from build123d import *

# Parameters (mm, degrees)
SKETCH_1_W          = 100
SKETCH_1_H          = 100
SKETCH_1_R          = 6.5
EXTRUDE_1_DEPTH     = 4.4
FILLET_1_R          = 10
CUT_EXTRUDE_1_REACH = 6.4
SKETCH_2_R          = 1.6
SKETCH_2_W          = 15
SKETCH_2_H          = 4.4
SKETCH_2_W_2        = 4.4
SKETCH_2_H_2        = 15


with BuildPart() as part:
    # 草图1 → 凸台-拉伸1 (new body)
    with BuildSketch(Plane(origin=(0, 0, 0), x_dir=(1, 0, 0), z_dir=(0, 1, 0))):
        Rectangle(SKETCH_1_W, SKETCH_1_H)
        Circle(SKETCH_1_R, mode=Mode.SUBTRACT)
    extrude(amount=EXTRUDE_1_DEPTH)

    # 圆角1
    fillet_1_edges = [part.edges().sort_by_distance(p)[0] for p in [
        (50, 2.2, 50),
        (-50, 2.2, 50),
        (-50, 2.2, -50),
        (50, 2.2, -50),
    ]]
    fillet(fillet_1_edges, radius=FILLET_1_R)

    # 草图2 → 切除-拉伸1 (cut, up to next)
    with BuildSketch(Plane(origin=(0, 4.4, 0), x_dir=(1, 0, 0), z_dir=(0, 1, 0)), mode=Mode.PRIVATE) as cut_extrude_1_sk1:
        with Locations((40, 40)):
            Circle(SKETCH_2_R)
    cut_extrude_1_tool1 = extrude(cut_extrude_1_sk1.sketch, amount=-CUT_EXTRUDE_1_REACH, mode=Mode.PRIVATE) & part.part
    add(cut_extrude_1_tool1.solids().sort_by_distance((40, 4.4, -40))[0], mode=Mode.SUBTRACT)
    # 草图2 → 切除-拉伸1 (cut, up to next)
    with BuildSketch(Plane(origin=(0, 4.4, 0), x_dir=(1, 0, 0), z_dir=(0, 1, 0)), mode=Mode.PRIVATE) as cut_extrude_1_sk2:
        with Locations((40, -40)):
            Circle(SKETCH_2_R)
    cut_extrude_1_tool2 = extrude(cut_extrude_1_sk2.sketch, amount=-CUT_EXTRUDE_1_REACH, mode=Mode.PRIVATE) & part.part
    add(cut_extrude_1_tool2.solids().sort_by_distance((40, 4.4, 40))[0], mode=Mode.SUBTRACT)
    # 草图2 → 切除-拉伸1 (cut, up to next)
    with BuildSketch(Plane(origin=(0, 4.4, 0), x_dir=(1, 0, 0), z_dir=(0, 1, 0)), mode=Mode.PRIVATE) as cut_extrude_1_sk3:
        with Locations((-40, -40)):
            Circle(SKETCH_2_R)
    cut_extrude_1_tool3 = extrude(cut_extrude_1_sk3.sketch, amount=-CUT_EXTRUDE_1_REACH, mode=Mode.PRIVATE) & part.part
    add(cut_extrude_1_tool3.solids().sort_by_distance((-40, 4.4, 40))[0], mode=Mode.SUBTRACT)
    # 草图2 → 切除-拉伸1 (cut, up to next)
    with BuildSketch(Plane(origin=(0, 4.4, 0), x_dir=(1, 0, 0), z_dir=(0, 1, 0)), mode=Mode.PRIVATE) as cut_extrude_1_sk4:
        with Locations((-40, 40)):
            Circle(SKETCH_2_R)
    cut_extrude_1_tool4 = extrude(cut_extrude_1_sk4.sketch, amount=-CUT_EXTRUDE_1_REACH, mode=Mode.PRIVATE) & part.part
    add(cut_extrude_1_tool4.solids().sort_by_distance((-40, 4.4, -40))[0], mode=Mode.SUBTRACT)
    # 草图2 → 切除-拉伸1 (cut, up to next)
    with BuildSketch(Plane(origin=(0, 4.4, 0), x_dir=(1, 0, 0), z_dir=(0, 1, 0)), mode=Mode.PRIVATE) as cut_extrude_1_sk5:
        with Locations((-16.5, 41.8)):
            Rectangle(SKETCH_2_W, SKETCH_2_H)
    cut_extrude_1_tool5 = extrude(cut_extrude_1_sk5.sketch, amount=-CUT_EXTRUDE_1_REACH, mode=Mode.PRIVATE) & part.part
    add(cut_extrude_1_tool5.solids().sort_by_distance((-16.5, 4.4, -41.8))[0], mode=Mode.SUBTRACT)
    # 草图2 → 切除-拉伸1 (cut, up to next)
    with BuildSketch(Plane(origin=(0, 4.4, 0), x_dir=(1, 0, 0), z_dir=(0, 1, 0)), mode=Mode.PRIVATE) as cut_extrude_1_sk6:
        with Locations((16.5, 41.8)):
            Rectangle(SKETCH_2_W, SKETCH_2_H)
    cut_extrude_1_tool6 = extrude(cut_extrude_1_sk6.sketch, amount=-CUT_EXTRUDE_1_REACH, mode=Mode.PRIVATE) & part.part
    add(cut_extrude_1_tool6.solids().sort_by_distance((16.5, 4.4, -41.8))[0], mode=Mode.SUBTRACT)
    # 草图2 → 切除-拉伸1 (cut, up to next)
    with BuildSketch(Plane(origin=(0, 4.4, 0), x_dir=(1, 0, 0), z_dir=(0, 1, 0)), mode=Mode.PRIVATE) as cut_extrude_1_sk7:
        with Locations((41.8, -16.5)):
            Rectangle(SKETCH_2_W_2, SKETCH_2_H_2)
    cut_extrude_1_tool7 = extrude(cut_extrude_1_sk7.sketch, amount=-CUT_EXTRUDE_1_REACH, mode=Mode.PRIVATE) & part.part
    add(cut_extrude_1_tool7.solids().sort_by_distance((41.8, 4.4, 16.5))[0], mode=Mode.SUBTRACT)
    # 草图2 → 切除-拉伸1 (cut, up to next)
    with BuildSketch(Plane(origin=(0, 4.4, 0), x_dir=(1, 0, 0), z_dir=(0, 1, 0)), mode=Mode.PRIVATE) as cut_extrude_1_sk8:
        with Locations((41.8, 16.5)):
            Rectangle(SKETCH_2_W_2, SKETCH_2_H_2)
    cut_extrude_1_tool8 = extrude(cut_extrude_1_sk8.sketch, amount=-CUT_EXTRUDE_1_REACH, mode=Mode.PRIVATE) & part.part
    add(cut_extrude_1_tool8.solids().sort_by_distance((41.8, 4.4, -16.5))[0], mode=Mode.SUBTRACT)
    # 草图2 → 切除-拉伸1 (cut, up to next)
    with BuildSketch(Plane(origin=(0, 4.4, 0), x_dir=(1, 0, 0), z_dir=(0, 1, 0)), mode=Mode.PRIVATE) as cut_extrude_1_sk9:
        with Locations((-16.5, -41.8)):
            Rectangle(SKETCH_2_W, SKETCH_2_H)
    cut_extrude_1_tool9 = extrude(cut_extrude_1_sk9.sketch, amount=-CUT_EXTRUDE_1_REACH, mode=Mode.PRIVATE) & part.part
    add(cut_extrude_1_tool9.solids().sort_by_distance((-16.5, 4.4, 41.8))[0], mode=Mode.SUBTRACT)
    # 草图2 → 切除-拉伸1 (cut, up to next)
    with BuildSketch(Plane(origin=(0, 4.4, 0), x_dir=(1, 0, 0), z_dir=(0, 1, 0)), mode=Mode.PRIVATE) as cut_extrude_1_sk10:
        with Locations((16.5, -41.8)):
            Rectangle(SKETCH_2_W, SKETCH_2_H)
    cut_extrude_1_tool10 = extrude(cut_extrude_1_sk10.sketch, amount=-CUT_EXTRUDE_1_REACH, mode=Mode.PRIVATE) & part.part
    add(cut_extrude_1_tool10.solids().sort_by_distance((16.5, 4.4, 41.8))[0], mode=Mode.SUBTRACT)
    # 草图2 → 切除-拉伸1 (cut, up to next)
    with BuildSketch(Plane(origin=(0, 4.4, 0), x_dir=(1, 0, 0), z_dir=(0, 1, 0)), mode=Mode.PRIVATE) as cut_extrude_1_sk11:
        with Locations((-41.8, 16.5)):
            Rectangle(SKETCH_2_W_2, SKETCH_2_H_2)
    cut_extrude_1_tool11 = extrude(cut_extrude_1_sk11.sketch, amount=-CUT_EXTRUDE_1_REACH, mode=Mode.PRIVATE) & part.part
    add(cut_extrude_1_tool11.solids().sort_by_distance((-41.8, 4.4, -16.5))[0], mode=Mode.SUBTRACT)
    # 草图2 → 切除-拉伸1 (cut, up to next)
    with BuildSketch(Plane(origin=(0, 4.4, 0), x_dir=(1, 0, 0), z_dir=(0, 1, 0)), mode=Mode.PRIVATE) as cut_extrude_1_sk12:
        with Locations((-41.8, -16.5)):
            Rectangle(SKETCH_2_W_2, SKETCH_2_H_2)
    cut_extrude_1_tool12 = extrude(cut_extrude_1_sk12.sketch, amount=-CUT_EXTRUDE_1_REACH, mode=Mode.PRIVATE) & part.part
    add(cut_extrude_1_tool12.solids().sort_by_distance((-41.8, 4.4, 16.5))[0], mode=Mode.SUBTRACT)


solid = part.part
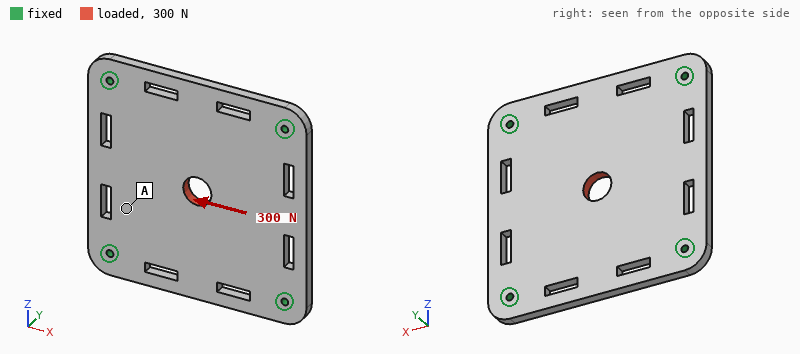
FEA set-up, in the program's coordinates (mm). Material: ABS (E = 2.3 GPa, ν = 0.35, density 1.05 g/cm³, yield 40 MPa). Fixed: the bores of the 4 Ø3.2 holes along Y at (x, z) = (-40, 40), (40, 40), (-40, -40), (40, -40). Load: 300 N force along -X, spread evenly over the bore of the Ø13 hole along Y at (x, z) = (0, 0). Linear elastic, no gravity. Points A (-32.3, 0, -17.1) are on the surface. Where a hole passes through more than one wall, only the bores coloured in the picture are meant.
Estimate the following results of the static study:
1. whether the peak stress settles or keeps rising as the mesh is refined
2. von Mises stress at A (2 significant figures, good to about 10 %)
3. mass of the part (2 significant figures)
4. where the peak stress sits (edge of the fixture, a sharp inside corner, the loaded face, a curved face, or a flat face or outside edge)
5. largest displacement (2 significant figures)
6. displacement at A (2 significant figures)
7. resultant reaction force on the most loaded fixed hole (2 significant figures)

keeps rising
0.64 MPa
43 g
edge of the fixture
31 µm
17 µm
84 N
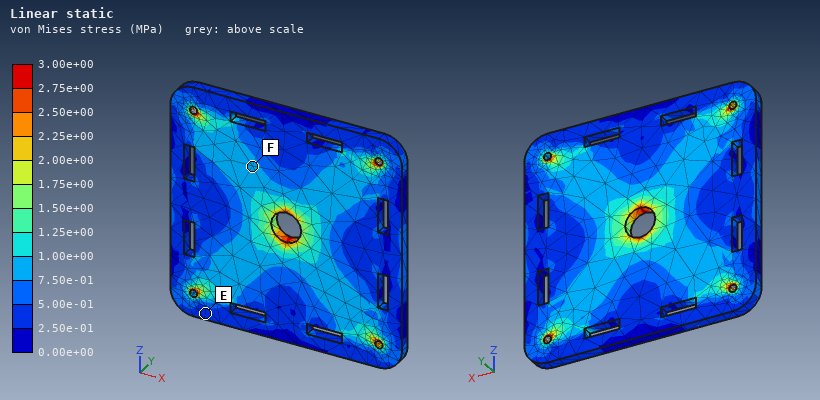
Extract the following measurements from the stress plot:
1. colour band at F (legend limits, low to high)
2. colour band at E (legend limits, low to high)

7.50e-01 to 1.00e+00 MPa
2.50e-01 to 5.00e-01 MPa
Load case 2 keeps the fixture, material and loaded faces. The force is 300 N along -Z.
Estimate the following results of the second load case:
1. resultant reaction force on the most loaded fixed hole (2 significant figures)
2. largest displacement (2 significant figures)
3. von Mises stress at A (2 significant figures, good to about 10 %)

84 N
31 µm
0.71 MPa
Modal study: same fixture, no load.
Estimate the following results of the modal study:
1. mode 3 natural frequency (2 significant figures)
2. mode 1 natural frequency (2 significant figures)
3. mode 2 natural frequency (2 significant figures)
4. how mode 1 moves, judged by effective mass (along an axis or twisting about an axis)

1100 Hz
650 Hz
1100 Hz
along Y
